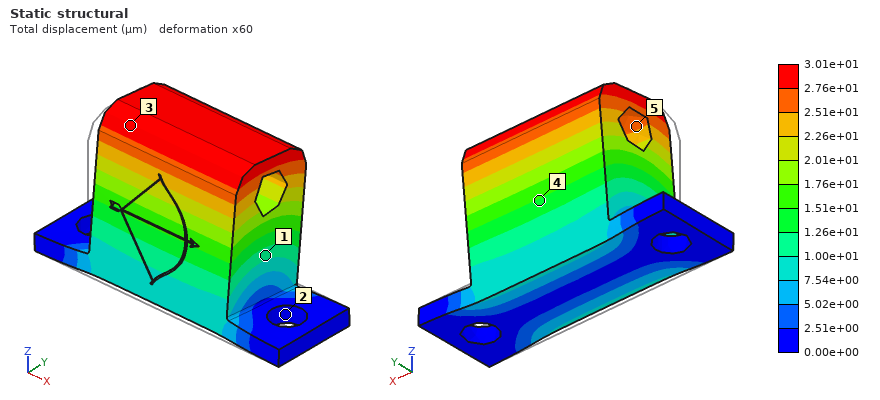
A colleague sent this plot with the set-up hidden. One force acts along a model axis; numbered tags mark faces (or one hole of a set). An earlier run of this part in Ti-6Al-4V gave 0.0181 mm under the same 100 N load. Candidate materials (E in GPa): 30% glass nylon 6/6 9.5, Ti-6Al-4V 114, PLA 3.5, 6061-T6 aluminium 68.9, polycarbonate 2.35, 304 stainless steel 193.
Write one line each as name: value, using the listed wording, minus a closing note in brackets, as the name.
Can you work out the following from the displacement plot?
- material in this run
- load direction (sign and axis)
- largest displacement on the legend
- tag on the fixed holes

material in this run: 6061-T6 aluminium
load direction: +Y
largest displacement on the legend: 3.01e+01 µm
tag on the fixed holes: 2
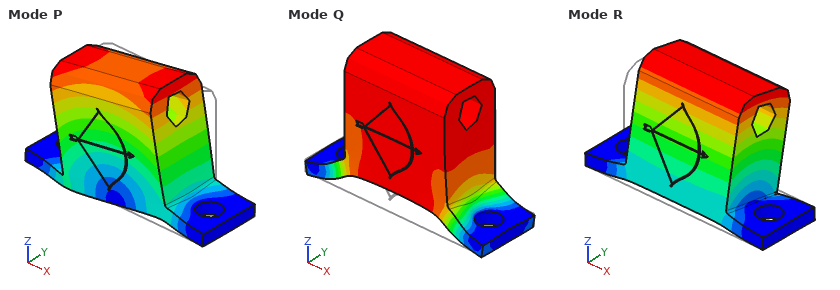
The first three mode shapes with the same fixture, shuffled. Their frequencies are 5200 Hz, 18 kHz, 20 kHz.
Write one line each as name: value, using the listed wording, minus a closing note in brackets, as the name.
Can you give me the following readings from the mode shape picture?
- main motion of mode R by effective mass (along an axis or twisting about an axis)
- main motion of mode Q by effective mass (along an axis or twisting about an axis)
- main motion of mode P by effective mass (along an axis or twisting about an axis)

main motion of mode R by effective mass: along Y
main motion of mode Q by effective mass: along Z
main motion of mode P by effective mass: along X
